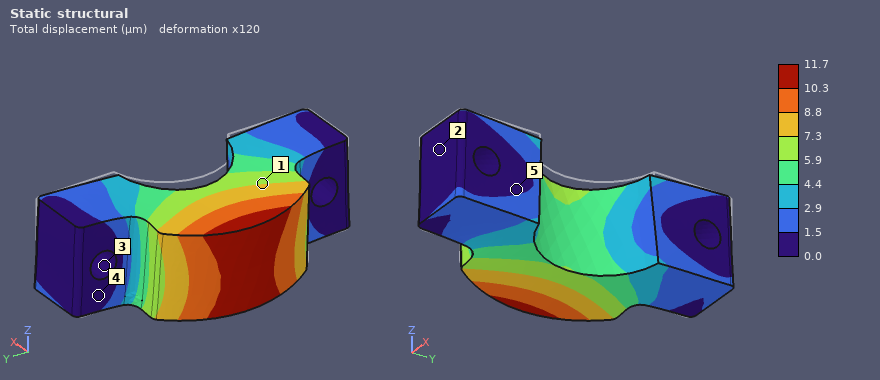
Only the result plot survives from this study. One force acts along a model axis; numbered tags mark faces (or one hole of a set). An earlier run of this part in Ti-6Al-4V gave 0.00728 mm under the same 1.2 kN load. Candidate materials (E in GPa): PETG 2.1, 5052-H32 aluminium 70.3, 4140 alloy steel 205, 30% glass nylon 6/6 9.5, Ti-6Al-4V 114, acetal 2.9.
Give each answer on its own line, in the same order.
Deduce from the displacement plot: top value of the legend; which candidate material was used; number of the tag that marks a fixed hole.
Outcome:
11.7 µm
5052-H32 aluminium
3
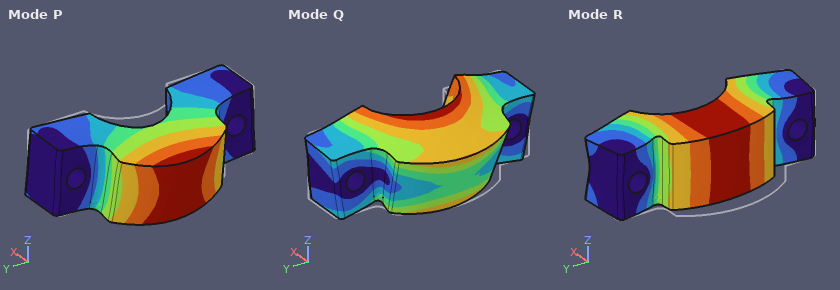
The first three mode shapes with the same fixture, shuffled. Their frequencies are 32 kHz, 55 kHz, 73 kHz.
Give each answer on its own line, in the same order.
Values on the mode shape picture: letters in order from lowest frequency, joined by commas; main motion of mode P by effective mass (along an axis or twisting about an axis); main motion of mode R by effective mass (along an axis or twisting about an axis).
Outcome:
P, R, Q
along Z
along X
